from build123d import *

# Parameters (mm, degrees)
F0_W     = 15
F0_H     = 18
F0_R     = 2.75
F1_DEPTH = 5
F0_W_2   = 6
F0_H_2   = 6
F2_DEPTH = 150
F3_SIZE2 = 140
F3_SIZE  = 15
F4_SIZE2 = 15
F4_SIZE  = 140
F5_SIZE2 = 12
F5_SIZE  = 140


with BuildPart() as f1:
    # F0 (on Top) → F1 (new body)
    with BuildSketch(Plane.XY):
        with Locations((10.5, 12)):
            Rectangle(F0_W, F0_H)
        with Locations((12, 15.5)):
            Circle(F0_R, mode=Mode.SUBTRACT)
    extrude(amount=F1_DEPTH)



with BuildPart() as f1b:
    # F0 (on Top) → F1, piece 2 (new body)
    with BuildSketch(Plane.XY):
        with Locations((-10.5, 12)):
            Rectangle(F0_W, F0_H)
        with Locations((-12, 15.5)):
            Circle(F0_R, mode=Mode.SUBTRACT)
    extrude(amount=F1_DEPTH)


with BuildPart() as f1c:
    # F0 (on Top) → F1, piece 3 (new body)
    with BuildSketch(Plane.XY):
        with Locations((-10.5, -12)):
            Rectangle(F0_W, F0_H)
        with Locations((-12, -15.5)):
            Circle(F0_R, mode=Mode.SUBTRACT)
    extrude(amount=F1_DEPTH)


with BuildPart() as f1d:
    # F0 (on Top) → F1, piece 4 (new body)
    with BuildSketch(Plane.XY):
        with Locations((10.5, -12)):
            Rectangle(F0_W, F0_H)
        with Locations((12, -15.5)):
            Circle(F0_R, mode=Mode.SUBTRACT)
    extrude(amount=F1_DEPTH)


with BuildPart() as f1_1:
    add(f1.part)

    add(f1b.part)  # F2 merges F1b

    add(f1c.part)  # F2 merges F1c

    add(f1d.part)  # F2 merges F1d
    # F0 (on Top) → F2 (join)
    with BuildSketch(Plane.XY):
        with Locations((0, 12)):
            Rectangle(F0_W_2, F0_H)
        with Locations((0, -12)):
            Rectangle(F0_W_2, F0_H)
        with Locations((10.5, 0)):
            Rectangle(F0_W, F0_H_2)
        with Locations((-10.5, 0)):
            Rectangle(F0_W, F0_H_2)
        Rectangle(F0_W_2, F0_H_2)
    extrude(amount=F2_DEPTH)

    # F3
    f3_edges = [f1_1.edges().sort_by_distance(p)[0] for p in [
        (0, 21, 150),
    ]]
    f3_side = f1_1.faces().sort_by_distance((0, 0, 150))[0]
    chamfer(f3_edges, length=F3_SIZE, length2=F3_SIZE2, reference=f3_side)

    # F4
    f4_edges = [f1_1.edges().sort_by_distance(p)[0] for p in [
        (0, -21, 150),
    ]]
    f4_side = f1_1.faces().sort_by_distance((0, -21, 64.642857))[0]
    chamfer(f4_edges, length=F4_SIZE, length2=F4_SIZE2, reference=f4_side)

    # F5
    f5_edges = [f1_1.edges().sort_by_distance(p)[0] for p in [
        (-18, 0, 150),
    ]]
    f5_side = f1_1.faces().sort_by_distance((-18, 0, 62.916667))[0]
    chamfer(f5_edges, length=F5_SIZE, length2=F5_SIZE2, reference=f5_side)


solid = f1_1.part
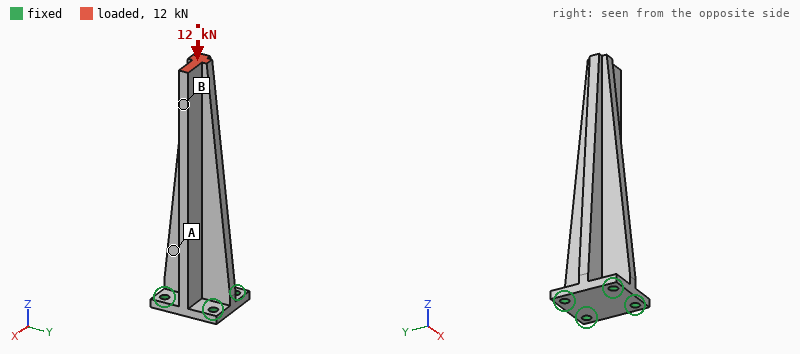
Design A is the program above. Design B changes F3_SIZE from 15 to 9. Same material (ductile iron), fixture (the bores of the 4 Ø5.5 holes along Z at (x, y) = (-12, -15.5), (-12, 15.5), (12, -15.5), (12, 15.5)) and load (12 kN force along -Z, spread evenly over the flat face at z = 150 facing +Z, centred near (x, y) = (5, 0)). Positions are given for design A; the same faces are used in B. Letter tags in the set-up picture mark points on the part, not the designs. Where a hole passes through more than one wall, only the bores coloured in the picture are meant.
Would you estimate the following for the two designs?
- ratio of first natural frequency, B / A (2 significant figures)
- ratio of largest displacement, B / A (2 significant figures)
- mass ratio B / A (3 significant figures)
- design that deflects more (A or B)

0.95
0.84
1.05
A
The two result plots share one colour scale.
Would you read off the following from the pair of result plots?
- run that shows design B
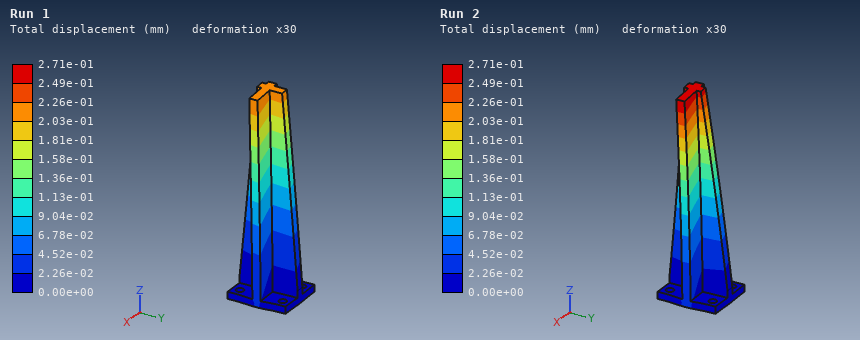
Run 1
